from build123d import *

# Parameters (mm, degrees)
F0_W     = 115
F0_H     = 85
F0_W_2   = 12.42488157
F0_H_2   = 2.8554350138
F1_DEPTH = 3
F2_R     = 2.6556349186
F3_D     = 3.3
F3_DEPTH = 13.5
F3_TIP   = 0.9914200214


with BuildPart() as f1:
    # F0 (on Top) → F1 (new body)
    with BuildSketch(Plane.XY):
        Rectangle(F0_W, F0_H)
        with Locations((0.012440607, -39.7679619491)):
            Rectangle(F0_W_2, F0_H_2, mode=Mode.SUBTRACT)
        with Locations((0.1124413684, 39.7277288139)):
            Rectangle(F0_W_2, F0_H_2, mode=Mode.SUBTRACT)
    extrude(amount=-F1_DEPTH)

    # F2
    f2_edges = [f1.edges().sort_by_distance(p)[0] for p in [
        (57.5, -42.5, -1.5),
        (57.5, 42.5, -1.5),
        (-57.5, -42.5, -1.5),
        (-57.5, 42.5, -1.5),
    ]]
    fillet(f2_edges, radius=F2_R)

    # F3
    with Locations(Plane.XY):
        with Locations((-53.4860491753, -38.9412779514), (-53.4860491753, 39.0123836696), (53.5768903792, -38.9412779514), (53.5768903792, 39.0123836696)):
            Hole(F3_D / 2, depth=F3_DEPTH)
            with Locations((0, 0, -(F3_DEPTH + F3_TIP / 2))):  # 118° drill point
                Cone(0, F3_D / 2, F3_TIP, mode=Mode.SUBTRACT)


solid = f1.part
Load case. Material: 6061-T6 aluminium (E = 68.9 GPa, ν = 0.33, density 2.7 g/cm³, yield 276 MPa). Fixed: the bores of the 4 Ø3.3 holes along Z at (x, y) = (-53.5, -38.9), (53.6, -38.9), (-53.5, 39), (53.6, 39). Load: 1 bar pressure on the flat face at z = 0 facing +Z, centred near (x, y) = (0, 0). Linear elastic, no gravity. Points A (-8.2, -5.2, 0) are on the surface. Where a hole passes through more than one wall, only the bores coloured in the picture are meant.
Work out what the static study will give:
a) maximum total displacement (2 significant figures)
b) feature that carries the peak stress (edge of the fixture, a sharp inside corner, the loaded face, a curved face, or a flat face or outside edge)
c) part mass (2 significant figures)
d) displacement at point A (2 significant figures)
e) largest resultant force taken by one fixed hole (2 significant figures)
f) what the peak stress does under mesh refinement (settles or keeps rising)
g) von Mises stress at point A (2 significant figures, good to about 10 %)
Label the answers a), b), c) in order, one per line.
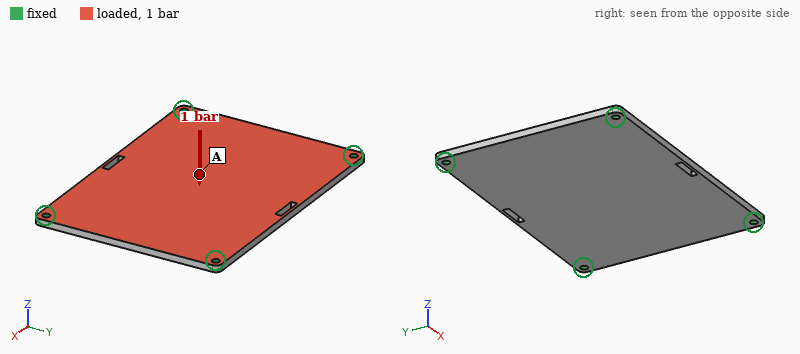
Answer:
a) 0.44 mm
b) edge of the fixture
c) 78 g
d) 0.43 mm
e) 240 N
f) keeps rising
g) 37 MPa
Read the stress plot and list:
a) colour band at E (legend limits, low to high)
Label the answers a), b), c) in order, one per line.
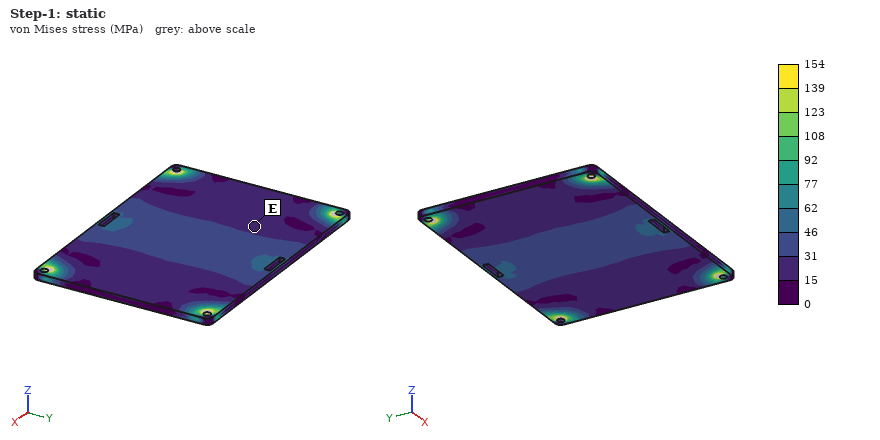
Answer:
a) 15 to 31 MPa
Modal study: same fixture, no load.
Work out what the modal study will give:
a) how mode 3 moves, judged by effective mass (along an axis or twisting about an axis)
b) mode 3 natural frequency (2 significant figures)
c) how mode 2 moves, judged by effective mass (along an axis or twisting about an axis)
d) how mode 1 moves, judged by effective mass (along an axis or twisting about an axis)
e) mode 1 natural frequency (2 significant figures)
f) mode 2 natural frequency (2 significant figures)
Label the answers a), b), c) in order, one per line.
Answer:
a) twisting about Y
b) 2300 Hz
c) twisting about X
d) along Z
e) 980 Hz
f) 1700 Hz
